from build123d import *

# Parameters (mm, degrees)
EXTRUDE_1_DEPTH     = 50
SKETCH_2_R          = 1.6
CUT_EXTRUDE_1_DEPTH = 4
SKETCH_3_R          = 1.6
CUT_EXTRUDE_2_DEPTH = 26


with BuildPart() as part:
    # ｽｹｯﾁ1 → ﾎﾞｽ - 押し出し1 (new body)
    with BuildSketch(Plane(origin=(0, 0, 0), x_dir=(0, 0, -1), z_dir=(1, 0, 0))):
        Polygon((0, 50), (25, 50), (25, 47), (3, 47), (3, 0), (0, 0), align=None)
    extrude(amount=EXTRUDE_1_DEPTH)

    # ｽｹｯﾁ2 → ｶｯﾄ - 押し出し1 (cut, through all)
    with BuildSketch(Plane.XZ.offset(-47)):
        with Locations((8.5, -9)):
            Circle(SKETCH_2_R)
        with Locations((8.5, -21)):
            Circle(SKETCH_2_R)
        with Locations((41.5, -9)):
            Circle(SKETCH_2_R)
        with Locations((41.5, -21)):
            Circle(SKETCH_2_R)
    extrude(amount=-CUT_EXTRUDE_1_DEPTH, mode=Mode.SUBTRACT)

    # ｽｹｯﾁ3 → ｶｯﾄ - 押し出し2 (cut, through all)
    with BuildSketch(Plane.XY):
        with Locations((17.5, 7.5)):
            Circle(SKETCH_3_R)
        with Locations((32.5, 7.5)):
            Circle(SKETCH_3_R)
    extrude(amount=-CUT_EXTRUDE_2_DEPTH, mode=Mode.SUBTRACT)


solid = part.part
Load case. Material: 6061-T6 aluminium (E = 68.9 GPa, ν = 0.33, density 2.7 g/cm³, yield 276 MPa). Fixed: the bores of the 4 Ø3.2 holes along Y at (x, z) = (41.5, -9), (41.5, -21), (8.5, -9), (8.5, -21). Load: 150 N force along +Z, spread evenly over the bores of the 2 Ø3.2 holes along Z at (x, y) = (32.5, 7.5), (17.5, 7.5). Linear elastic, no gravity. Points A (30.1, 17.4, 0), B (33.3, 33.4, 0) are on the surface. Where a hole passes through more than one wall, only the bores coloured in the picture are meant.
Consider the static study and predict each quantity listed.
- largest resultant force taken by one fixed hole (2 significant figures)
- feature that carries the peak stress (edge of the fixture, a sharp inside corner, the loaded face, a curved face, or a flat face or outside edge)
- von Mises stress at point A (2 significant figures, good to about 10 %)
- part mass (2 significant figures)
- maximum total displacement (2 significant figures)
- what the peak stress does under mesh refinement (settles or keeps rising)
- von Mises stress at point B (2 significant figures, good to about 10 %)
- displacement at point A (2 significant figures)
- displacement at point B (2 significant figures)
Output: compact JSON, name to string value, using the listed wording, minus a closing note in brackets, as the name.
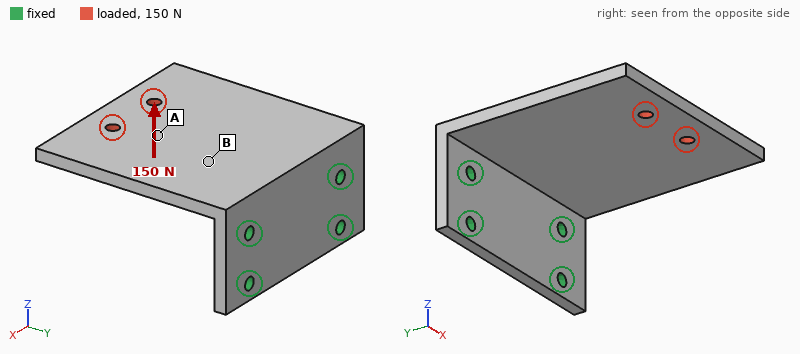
{"largest resultant force taken by one fixed hole": "120 N", "feature that carries the peak stress": "edge of the fixture", "von Mises stress at point A": "21 MPa", "part mass": "29 g", "maximum total displacement": "0.81 mm", "what the peak stress does under mesh refinement": "keeps rising", "von Mises stress at point B": "47 MPa", "displacement at point A": "0.45 mm", "displacement at point B": "0.16 mm"}
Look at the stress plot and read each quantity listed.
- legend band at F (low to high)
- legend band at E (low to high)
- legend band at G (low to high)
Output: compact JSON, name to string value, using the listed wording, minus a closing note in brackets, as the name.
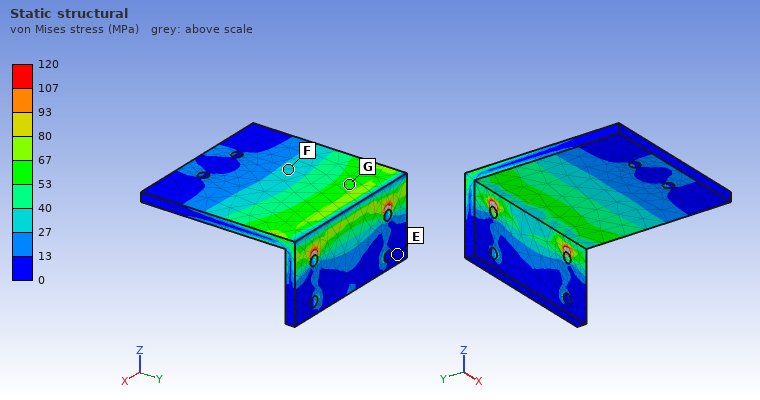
{"legend band at F": "27 to 40 MPa", "legend band at E": "0 to 13 MPa", "legend band at G": "53 to 67 MPa"}
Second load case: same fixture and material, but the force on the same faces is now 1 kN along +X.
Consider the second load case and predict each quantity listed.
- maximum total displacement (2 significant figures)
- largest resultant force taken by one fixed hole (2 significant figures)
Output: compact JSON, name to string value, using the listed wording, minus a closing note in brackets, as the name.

{"maximum total displacement": "0.23 mm", "largest resultant force taken by one fixed hole": "1.4 kN"}
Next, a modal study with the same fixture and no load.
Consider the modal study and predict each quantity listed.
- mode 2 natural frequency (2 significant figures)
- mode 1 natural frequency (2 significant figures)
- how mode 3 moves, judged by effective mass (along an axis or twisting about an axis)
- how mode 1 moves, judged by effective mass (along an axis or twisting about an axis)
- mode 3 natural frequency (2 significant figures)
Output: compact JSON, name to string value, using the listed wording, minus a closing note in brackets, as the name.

{"mode 2 natural frequency": "2200 Hz", "mode 1 natural frequency": "860 Hz", "how mode 3 moves, judged by effective mass": "along X", "how mode 1 moves, judged by effective mass": "along Z", "mode 3 natural frequency": "4300 Hz"}
